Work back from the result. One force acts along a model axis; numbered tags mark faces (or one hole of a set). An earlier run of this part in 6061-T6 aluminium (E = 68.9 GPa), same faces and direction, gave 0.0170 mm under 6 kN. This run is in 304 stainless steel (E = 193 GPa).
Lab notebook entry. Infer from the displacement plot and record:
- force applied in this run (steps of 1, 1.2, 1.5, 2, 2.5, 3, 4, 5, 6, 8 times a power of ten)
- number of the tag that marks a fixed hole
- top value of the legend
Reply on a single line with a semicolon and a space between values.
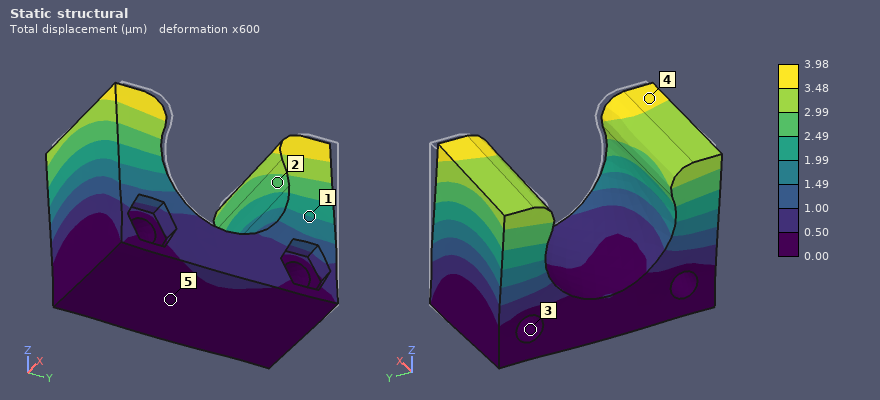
4 kN; 3; 3.98 µm
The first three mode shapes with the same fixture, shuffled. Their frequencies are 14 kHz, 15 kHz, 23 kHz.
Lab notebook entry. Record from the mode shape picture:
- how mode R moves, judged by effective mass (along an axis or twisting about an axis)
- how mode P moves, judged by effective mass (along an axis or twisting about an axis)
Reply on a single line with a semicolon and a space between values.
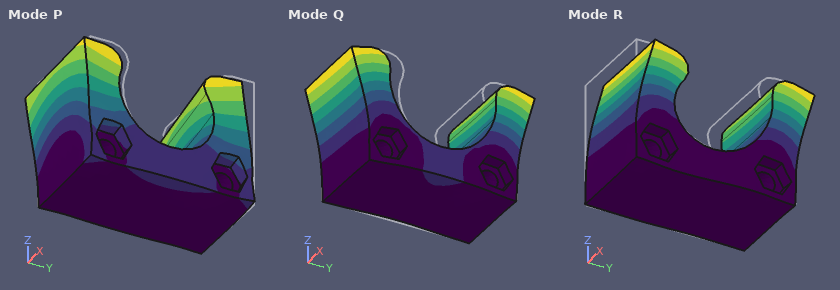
along Y; along X
